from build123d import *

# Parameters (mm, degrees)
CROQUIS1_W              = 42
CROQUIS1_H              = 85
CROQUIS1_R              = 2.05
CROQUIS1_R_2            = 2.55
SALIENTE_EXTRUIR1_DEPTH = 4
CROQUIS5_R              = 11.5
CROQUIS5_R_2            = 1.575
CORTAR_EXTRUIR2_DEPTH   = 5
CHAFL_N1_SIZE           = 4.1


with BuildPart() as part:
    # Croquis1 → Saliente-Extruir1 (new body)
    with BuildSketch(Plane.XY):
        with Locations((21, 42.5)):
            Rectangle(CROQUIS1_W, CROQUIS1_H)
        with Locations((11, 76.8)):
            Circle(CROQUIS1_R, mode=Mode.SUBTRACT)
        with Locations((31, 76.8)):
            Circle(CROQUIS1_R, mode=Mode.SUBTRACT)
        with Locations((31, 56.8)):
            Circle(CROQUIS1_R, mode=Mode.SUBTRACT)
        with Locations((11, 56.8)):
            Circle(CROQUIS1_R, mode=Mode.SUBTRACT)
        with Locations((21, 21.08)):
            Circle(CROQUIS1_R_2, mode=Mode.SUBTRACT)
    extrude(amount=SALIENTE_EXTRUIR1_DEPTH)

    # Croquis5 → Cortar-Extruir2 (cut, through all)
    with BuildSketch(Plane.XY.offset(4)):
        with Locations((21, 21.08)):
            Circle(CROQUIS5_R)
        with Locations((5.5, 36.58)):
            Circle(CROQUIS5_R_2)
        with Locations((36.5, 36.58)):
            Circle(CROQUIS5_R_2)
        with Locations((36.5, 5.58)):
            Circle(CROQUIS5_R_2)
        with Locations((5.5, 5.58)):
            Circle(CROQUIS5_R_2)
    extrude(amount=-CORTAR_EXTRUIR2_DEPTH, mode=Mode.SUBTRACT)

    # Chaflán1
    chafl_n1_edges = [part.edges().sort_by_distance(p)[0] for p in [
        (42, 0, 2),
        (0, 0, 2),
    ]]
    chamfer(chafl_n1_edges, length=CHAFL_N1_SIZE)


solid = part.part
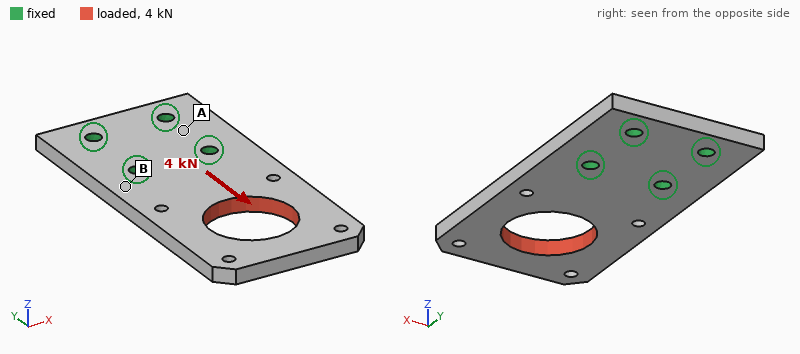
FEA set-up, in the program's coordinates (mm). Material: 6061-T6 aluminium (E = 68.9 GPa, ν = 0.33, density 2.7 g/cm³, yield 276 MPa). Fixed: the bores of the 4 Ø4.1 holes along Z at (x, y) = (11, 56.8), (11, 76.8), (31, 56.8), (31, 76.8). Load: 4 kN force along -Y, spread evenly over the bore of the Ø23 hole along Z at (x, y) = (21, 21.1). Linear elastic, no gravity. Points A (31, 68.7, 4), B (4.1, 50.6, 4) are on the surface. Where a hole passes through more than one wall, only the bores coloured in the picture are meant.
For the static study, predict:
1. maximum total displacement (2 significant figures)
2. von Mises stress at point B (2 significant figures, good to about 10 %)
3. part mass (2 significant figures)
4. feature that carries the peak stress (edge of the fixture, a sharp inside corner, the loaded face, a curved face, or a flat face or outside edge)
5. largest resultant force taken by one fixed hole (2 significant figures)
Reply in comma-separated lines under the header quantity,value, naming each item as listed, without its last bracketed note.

quantity,value
maximum total displacement,35 µm
von Mises stress at point B,24 MPa
part mass,33 g
feature that carries the peak stress,a curved face
largest resultant force taken by one fixed hole,1.7 kN
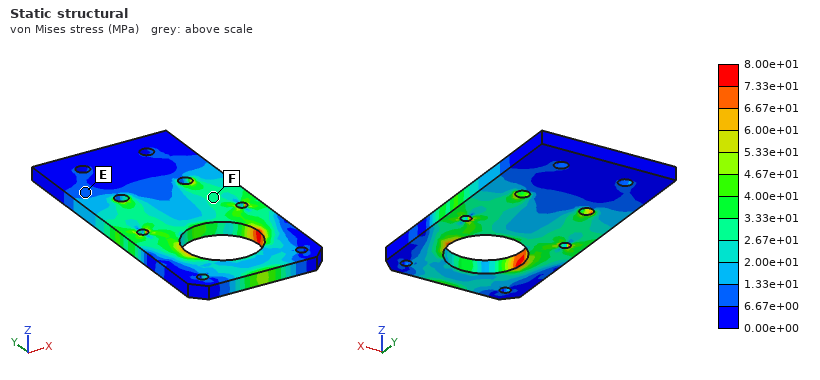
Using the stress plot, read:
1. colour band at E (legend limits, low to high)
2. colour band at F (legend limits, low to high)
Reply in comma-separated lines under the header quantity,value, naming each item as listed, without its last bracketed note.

quantity,value
colour band at E,6.67e+00 to 1.33e+01 MPa
colour band at F,2.67e+01 to 3.33e+01 MPa
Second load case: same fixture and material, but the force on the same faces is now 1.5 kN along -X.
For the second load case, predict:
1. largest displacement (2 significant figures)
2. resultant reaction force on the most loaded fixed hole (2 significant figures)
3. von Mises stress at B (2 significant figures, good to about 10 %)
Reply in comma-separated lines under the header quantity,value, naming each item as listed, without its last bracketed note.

quantity,value
largest displacement,83 µm
resultant reaction force on the most loaded fixed hole,1.8 kN
von Mises stress at B,26 MPa
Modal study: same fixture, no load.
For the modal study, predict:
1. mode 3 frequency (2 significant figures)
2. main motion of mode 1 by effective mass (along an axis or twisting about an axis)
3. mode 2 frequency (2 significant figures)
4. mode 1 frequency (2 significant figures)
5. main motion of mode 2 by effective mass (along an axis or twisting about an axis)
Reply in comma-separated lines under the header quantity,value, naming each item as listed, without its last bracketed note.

quantity,value
mode 3 frequency,5700 Hz
main motion of mode 1 by effective mass,along Z
mode 2 frequency,2800 Hz
mode 1 frequency,1100 Hz
main motion of mode 2 by effective mass,twisting about Y
